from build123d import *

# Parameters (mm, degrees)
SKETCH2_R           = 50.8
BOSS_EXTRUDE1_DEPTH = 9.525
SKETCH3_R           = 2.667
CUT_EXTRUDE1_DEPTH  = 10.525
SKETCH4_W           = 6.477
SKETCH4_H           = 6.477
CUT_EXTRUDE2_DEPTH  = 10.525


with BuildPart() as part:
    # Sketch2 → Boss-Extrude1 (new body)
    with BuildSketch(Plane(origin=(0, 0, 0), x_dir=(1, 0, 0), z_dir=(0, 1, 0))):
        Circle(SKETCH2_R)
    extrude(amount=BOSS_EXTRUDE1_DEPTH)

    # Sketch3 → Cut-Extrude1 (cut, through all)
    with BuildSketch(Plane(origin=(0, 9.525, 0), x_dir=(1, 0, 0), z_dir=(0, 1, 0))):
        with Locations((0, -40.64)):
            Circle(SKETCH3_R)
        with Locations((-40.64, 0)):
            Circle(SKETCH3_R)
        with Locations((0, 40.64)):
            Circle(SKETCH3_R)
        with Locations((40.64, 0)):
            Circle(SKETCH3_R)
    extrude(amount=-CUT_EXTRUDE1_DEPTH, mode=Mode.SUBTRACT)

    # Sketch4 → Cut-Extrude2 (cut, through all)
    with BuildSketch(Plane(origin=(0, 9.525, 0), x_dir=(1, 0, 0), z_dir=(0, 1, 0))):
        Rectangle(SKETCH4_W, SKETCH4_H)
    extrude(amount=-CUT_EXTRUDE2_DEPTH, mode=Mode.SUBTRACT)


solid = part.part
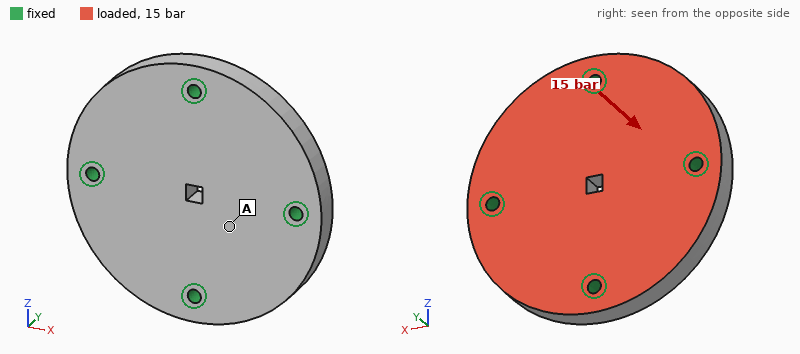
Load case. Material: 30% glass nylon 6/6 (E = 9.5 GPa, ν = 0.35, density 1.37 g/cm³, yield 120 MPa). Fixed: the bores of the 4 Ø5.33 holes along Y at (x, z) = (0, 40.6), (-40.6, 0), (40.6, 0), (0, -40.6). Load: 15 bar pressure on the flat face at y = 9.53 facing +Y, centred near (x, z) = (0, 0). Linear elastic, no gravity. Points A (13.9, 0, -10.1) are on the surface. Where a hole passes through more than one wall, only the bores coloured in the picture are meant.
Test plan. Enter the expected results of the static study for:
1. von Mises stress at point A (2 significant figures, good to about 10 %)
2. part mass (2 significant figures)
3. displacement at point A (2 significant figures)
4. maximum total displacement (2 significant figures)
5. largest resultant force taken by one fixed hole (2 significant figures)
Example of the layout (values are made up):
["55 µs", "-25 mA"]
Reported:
["13 MPa", "100 g", "0.15 mm", "0.18 mm", "3.0 kN"]
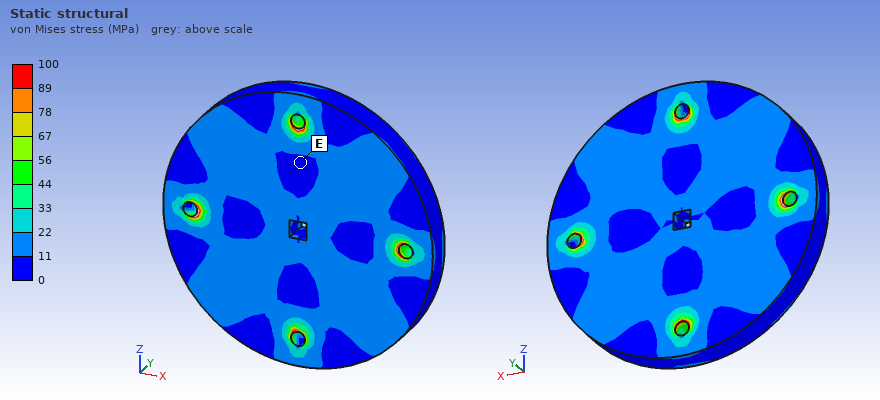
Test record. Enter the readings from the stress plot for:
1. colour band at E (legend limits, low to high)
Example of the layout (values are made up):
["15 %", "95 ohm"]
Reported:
["0 to 11 MPa"]
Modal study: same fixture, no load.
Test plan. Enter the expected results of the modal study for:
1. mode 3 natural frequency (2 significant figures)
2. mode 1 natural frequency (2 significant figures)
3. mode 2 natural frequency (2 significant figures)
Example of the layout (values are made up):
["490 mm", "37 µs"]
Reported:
["5100 Hz", "4800 Hz", "4800 Hz"]
